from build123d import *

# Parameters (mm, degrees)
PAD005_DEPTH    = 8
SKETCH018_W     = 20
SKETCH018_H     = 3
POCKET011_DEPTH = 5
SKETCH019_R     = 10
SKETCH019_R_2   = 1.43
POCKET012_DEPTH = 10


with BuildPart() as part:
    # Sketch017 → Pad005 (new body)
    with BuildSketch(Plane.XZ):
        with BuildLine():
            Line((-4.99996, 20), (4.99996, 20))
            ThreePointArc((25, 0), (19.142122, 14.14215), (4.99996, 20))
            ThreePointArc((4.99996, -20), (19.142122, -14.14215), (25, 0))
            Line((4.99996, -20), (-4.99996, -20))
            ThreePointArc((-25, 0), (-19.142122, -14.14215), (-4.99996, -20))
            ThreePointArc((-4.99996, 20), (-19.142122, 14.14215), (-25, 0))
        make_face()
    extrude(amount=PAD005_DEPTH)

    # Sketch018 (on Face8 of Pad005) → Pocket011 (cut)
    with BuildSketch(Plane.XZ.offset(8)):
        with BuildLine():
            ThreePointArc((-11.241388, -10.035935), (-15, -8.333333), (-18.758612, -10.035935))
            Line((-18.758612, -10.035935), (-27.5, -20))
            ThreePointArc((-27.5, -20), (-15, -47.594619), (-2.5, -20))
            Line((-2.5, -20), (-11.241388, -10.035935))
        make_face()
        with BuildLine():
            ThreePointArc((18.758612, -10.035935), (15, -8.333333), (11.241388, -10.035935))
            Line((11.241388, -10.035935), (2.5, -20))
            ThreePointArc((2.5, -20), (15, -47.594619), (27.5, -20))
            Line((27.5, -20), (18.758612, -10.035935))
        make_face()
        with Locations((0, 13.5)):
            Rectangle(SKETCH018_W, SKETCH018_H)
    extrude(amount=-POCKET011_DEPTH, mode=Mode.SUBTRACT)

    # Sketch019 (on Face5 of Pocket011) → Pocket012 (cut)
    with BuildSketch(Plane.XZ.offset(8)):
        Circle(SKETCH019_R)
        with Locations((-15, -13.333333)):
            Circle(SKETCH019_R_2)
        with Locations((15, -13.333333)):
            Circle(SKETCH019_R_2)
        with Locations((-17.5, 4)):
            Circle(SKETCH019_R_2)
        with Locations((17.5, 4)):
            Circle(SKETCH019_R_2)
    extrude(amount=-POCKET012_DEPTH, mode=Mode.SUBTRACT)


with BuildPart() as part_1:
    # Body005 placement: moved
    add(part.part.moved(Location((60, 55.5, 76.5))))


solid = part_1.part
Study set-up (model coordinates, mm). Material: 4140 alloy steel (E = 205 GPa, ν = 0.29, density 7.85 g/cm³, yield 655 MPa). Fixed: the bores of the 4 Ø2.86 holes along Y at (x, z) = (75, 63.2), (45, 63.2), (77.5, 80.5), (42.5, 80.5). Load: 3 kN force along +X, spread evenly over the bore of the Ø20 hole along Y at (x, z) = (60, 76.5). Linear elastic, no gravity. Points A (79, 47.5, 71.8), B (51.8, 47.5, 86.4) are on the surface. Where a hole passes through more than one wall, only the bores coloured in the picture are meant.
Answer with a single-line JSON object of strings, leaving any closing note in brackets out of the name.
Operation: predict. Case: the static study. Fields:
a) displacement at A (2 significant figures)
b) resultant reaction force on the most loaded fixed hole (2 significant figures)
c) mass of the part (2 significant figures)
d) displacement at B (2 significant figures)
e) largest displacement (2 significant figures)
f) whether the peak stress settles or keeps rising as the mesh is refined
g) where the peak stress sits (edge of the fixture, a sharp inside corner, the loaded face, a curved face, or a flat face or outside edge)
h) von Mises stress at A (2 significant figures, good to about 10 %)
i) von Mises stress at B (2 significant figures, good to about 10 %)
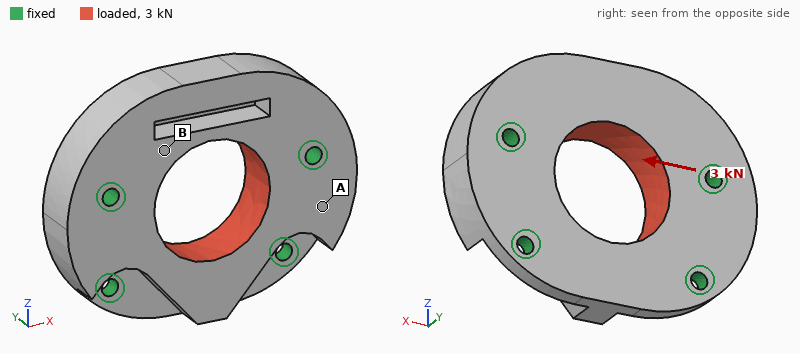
{"displacement at A": "0.45 µm", "resultant reaction force on the most loaded fixed hole": "1.1 kN", "mass of the part": "72 g", "displacement at B": "0.72 µm", "largest displacement": "1.0 µm", "whether the peak stress settles or keeps rising as the mesh is refined": "keeps rising", "where the peak stress sits": "edge of the fixture", "von Mises stress at A": "3.5 MPa", "von Mises stress at B": "8.9 MPa"}
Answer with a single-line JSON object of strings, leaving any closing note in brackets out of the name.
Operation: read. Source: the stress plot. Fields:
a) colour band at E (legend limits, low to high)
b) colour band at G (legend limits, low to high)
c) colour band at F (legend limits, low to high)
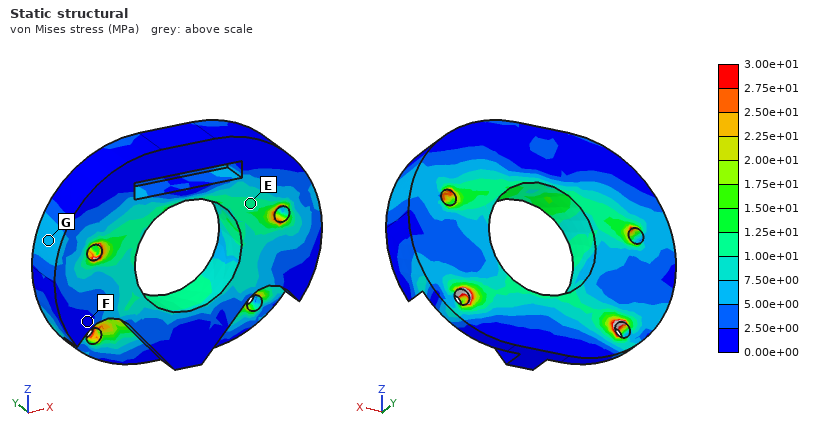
{"colour band at E": "1.00e+01 to 1.25e+01 MPa", "colour band at G": "5.00e+00 to 7.50e+00 MPa", "colour band at F": "0.00e+00 to 2.50e+00 MPa"}
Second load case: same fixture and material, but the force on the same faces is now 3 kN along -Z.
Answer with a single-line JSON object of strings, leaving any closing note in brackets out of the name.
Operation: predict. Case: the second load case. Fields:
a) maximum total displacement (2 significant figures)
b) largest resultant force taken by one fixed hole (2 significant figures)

{"maximum total displacement": "3.3 µm", "largest resultant force taken by one fixed hole": "1.1 kN"}
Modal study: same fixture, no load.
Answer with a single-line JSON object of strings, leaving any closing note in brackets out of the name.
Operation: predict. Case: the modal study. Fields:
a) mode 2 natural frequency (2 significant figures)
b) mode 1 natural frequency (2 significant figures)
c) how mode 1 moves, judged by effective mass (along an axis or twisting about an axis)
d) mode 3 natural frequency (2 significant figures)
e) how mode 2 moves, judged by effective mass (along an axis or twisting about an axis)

{"mode 2 natural frequency": "20 kHz", "mode 1 natural frequency": "16 kHz", "how mode 1 moves, judged by effective mass": "along Y", "mode 3 natural frequency": "30 kHz", "how mode 2 moves, judged by effective mass": "along Y"}
